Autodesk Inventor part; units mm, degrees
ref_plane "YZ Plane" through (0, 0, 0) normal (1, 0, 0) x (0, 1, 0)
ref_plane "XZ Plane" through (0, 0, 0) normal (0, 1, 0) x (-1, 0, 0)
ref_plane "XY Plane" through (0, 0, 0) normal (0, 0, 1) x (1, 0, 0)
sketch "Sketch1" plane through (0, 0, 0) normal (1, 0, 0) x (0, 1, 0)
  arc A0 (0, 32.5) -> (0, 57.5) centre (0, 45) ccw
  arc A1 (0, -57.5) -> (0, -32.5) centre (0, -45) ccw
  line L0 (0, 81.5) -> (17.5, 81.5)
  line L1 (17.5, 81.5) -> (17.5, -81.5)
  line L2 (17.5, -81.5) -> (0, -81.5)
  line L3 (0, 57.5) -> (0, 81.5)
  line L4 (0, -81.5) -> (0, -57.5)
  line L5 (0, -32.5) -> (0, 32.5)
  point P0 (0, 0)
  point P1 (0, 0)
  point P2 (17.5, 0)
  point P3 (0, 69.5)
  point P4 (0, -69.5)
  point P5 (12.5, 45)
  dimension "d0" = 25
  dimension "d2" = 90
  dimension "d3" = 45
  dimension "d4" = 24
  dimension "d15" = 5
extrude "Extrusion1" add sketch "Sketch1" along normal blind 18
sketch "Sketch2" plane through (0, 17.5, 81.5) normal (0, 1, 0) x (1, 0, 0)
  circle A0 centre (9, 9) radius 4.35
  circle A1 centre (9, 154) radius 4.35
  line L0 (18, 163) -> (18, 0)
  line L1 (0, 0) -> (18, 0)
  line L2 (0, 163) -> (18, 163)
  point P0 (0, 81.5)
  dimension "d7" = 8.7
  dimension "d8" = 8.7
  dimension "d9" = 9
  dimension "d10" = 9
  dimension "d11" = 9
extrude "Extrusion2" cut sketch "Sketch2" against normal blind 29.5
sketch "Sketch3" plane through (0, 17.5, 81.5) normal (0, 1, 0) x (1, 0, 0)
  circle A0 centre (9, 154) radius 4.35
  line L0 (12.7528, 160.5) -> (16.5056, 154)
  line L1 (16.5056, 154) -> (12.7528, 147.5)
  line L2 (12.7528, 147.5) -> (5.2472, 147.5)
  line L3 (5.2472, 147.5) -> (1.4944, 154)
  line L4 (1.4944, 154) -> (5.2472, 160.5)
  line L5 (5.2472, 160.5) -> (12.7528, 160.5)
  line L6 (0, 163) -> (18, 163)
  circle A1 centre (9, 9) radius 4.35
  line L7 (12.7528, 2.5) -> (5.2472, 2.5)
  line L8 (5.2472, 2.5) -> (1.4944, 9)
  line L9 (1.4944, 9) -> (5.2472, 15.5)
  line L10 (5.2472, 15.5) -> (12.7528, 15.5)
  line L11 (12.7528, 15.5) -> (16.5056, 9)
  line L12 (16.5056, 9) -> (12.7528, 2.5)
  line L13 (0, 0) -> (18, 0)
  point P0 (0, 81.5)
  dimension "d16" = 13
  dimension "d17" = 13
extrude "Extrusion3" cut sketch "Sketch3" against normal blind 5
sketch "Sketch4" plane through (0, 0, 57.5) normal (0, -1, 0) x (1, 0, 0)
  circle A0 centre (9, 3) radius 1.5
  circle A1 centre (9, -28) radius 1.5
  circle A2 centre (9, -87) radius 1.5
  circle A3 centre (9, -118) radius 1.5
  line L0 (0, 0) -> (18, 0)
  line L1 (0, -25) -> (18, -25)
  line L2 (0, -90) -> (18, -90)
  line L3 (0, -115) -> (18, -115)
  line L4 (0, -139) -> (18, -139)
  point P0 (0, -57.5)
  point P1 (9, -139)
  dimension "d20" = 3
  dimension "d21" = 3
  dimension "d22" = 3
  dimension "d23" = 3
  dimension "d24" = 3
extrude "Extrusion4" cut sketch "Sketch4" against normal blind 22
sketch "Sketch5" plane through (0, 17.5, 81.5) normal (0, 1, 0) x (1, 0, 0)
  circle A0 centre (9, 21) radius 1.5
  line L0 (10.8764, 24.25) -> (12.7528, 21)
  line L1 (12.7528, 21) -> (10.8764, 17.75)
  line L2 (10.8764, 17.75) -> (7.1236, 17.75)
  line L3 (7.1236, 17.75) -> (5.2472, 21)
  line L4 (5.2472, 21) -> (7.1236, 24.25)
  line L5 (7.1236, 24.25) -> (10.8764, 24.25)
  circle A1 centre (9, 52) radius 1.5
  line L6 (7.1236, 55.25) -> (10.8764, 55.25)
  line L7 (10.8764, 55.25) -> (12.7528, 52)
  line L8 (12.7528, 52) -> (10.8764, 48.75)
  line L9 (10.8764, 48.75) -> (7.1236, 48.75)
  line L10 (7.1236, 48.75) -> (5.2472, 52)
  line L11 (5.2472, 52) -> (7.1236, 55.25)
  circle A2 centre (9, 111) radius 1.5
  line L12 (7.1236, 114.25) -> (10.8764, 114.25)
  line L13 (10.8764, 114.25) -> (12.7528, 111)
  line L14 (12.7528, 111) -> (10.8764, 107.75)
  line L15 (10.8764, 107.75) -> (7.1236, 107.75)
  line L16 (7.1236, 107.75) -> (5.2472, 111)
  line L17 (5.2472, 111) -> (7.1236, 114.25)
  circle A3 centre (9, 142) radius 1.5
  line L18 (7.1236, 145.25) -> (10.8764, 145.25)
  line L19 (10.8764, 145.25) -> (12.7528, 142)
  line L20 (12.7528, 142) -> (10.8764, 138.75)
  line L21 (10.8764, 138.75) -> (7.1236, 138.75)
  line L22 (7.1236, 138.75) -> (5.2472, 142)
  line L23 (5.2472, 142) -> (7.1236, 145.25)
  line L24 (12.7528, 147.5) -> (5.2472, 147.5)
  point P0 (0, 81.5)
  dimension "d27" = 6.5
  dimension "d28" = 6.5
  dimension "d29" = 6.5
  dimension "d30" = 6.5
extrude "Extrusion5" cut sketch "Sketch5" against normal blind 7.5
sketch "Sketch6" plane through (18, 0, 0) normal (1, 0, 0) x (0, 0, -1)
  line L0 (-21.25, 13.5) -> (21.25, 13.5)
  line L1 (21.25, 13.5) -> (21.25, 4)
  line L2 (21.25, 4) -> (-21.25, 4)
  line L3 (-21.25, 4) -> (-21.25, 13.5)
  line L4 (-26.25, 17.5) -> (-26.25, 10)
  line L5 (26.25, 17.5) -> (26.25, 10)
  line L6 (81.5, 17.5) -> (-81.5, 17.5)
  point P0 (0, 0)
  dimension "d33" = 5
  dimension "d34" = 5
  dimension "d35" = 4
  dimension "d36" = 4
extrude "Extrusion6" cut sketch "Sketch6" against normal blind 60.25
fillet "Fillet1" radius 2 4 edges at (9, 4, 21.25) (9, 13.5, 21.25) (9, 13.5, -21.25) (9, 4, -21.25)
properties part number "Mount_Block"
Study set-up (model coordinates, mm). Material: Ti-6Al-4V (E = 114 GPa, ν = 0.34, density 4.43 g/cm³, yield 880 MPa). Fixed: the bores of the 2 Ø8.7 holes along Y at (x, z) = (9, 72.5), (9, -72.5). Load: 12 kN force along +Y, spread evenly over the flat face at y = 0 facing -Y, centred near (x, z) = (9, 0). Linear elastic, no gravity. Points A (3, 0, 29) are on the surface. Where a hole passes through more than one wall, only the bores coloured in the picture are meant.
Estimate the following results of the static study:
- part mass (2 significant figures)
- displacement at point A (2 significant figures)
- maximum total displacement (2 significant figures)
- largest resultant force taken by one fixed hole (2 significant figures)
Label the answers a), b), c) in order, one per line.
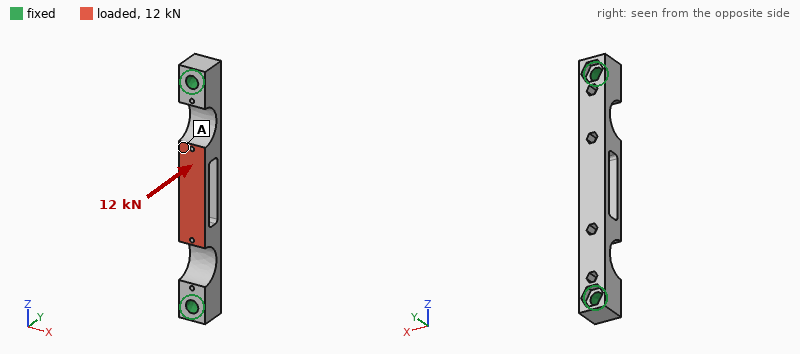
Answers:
a) 140 g
b) 0.32 mm
c) 0.60 mm
d) 6.2 kN
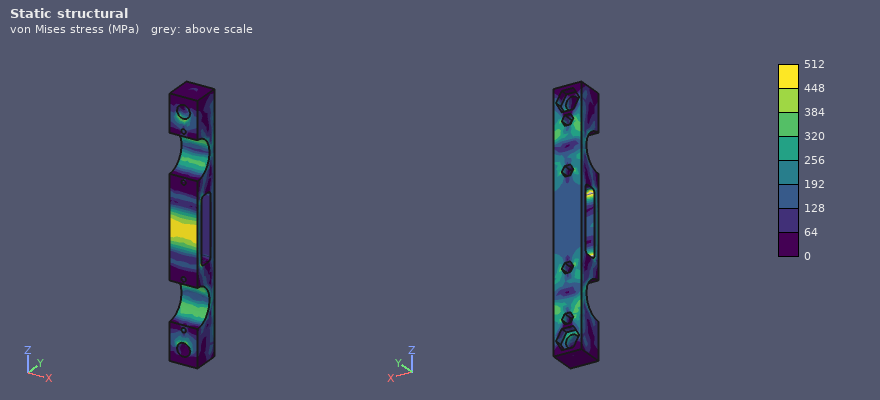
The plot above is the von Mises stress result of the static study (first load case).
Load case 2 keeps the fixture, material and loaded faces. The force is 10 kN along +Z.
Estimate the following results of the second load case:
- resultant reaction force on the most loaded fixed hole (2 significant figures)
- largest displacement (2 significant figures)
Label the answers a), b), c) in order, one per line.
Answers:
a) 5.2 kN
b) 0.12 mm
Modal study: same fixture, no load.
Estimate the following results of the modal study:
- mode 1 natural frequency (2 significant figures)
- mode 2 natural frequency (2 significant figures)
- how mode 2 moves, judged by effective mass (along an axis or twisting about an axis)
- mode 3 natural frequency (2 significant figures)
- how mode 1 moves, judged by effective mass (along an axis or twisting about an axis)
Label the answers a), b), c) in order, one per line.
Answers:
a) 3200 Hz
b) 3500 Hz
c) along Y
d) 4600 Hz
e) along X
